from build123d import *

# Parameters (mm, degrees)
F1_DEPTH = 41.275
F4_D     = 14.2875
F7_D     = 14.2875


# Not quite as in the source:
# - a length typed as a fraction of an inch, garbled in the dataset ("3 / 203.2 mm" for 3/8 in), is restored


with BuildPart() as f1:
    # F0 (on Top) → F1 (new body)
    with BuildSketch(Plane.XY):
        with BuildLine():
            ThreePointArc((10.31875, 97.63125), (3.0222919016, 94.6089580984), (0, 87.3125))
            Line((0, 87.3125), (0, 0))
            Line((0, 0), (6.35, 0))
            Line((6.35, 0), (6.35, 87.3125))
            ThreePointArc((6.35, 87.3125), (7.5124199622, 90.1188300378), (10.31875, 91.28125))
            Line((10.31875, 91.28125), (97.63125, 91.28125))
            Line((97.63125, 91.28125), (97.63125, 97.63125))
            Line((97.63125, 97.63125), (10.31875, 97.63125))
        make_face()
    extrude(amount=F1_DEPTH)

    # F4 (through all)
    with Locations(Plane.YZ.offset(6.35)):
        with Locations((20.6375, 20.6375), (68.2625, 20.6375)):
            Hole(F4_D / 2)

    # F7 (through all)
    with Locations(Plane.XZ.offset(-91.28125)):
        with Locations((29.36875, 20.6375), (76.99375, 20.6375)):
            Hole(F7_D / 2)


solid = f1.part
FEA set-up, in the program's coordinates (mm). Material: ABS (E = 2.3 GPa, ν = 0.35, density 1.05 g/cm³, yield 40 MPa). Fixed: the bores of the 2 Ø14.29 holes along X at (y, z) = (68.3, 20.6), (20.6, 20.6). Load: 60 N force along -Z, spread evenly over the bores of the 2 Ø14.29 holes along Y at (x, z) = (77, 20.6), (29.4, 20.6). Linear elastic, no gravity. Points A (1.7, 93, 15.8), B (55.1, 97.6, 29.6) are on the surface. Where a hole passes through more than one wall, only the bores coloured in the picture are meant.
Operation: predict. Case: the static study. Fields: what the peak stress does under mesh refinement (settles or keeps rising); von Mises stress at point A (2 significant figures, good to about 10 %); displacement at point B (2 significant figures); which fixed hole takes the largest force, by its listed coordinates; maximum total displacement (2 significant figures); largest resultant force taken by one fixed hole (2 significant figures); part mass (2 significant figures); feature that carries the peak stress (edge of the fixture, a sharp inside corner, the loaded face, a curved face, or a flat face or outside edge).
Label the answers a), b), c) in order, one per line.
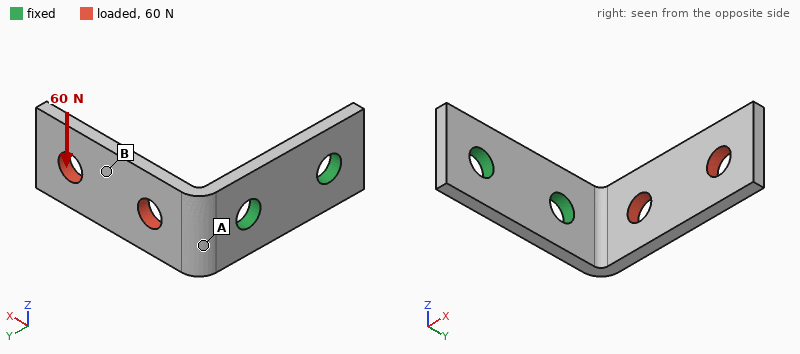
a) keeps rising
b) 4.4 MPa
c) 0.84 mm
d) (68.3, 20.6)
e) 1.6 mm
f) 73 N
g) 47 g
h) edge of the fixture
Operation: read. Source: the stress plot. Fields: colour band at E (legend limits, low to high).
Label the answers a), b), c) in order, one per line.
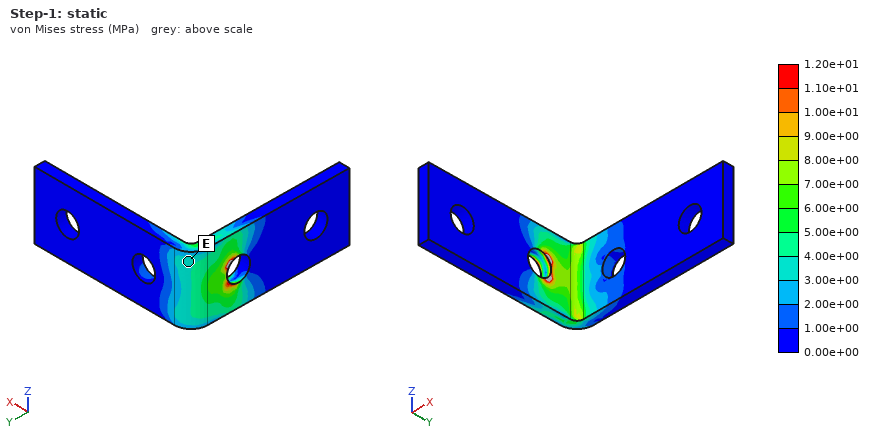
a) 3.00e+00 to 4.00e+00 MPa
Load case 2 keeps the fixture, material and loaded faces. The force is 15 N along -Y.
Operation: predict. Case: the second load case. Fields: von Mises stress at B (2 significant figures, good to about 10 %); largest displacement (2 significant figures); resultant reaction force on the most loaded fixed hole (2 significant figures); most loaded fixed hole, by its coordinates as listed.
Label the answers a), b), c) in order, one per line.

a) 0.63 MPa
b) 1.5 mm
c) 14 N
d) (68.3, 20.6)
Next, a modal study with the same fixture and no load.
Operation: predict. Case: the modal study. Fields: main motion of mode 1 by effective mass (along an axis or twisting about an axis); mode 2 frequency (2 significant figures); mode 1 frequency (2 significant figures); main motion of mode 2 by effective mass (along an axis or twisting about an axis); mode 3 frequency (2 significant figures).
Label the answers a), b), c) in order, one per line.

a) along Y
b) 250 Hz
c) 130 Hz
d) along Z
e) 700 Hz
